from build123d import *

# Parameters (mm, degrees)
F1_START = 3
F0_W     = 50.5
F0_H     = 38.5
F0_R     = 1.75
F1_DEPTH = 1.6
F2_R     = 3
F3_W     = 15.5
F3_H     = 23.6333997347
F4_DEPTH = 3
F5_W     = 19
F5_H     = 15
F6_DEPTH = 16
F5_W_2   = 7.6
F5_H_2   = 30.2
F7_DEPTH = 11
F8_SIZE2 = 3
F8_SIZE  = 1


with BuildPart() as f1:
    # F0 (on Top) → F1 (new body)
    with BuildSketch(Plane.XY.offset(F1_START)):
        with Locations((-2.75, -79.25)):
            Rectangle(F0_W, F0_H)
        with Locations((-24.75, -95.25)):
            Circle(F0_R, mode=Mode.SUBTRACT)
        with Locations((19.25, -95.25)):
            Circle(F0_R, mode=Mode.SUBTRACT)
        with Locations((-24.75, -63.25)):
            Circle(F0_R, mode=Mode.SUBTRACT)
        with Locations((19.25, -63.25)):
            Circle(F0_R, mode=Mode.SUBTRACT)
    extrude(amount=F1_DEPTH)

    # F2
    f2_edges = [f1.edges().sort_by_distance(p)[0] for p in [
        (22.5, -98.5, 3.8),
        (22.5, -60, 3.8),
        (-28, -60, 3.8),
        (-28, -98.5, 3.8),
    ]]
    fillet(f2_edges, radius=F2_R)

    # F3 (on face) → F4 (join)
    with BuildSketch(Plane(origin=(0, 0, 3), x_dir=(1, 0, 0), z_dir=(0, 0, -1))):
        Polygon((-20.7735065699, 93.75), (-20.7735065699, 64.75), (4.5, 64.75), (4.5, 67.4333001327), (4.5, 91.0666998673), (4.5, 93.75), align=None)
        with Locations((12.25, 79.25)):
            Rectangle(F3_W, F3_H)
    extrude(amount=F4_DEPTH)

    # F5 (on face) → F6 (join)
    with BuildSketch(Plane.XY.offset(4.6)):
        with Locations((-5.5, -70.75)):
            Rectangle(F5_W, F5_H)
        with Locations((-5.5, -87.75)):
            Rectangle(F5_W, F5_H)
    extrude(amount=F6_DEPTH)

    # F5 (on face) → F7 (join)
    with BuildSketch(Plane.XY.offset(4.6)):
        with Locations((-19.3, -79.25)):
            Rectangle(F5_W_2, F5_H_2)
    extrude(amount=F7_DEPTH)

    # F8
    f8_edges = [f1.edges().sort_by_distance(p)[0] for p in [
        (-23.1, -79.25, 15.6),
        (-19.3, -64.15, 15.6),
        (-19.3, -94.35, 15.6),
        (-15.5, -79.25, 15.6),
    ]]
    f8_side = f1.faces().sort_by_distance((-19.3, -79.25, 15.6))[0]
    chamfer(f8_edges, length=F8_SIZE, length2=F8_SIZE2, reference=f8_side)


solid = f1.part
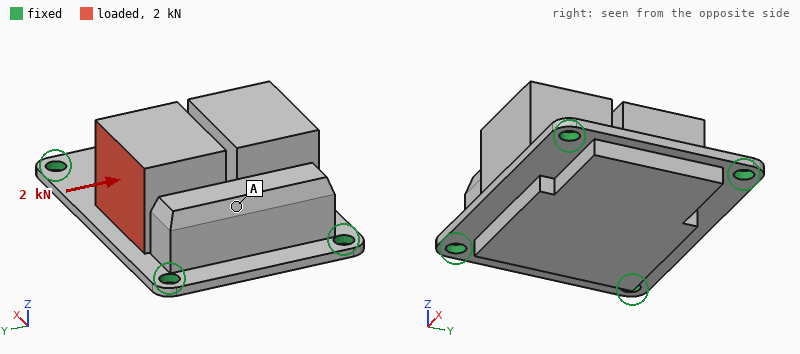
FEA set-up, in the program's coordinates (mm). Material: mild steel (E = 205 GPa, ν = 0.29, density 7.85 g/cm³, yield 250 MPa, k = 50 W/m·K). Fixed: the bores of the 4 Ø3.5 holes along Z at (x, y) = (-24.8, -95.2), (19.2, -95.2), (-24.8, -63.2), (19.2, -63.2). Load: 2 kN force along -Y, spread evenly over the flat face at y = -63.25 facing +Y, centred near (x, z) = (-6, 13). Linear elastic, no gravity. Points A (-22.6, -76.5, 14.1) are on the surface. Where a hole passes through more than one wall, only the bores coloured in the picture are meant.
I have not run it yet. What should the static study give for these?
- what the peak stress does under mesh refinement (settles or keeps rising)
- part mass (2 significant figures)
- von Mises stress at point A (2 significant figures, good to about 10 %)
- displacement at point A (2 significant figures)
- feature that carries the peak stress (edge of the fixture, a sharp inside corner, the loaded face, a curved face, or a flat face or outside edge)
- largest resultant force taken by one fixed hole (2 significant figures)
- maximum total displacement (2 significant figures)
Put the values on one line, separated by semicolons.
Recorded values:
keeps rising; 140 g; 17 MPa; 4.8 µm; edge of the fixture; 980 N; 27 µm
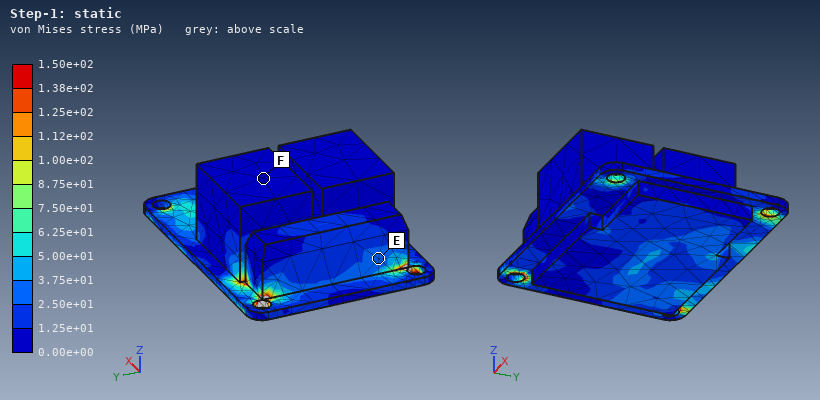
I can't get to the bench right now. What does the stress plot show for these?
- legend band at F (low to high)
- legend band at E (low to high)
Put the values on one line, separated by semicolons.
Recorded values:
0.00e+00 to 1.25e+01 MPa; 2.50e+01 to 3.75e+01 MPa
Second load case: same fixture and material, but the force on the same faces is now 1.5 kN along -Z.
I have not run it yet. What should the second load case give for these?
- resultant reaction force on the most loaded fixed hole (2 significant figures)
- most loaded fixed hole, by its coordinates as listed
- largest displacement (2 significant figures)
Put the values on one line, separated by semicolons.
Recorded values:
1.1 kN; (-24.8, -63.2); 41 µm
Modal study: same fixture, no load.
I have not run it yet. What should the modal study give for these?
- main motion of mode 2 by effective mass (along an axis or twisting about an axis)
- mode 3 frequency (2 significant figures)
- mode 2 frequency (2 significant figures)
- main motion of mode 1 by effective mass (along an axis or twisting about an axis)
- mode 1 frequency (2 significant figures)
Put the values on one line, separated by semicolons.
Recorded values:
along Y; 8700 Hz; 6400 Hz; along Z; 4400 Hz
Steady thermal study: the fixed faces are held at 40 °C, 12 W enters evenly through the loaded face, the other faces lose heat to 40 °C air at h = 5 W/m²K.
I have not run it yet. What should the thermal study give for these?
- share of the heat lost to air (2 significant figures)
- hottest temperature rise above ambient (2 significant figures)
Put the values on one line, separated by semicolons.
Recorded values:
5.7 %; 38 K
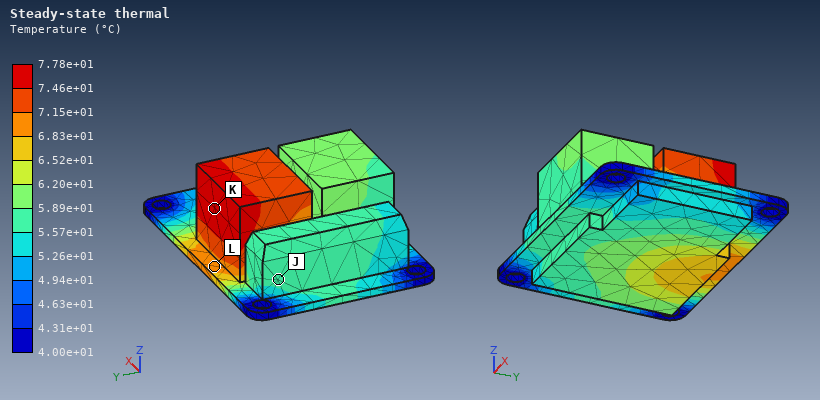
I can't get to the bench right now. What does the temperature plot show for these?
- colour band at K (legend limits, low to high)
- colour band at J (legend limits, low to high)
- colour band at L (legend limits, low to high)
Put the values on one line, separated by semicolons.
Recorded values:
7.46e+01 to 7.78e+01 °C; 5.57e+01 to 5.89e+01 °C; 6.83e+01 to 7.15e+01 °C
